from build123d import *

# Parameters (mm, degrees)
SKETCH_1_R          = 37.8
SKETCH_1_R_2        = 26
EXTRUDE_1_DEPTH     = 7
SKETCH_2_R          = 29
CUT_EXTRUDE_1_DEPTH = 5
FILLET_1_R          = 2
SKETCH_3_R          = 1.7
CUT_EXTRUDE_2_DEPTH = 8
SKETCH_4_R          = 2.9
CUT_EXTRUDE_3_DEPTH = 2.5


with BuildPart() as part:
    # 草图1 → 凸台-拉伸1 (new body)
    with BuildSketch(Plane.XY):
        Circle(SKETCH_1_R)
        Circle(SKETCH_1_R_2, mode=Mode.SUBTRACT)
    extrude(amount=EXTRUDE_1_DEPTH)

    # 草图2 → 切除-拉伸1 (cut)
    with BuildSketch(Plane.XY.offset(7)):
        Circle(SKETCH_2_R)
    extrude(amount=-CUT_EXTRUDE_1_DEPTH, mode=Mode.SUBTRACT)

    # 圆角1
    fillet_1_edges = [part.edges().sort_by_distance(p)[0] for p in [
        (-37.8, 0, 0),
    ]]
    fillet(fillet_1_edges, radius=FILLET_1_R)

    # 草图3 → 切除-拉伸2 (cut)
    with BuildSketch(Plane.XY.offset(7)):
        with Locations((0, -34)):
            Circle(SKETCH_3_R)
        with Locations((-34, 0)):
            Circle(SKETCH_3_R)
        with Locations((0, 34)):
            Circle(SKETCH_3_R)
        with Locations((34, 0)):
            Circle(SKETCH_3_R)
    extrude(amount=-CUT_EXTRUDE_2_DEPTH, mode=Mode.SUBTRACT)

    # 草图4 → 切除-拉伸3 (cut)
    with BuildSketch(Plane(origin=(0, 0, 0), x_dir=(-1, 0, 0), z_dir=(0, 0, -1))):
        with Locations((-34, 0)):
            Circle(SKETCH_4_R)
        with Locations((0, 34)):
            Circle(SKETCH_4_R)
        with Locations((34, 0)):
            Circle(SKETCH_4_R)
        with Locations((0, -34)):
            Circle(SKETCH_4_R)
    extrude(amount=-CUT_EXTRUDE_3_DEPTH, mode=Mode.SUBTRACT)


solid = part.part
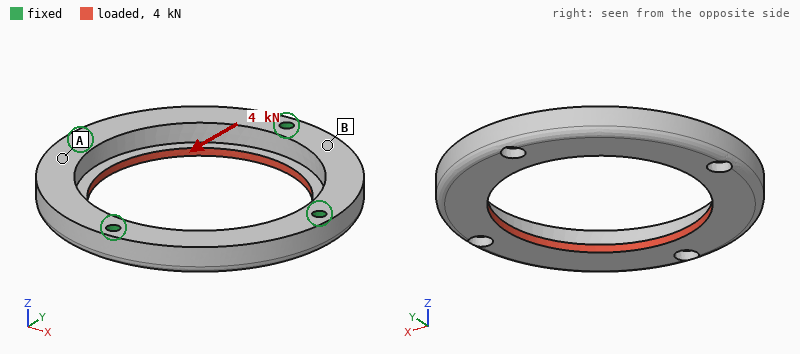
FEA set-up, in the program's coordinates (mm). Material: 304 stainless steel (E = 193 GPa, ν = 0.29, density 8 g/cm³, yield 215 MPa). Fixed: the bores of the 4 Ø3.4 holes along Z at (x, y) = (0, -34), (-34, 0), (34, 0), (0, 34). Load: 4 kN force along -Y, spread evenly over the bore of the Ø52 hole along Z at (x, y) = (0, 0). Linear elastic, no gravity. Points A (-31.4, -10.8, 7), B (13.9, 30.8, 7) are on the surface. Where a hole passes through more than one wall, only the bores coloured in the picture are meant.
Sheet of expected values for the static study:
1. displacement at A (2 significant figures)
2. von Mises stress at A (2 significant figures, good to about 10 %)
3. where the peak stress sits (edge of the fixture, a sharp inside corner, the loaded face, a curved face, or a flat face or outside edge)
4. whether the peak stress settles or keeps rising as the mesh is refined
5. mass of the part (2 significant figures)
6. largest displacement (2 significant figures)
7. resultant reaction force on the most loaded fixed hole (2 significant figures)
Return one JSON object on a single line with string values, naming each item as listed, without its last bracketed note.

{"displacement at A": "1.5 µm", "von Mises stress at A": "14 MPa", "where the peak stress sits": "edge of the fixture", "whether the peak stress settles or keeps rising as the mesh is refined": "keeps rising", "mass of the part": "110 g", "largest displacement": "4.9 µm", "resultant reaction force on the most loaded fixed hole": "1.3 kN"}
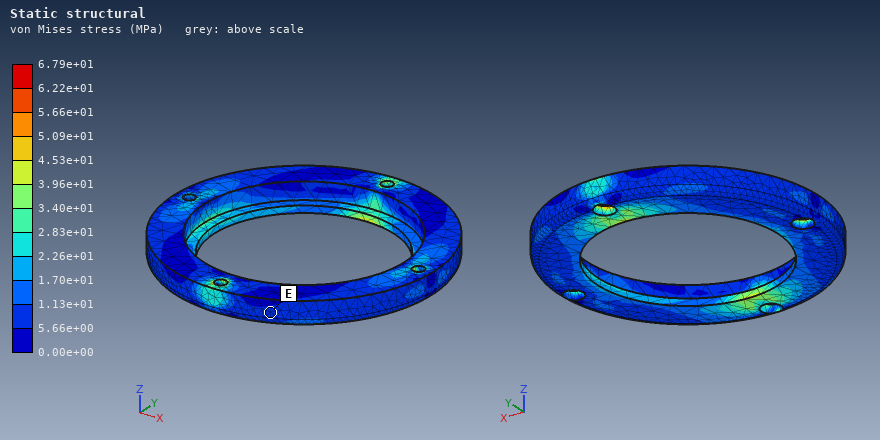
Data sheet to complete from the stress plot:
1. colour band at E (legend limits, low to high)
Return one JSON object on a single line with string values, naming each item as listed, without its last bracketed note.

{"colour band at E": "5.66e+00 to 1.13e+01 MPa"}
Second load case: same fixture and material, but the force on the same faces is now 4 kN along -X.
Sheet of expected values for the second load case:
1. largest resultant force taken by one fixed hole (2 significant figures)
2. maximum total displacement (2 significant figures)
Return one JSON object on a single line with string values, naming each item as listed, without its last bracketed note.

{"largest resultant force taken by one fixed hole": "1.3 kN", "maximum total displacement": "4.9 µm"}
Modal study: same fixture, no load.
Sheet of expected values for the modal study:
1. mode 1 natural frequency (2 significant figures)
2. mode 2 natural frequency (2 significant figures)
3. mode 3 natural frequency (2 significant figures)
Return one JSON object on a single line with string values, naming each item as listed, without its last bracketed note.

{"mode 1 natural frequency": "8300 Hz", "mode 2 natural frequency": "9400 Hz", "mode 3 natural frequency": "9400 Hz"}
